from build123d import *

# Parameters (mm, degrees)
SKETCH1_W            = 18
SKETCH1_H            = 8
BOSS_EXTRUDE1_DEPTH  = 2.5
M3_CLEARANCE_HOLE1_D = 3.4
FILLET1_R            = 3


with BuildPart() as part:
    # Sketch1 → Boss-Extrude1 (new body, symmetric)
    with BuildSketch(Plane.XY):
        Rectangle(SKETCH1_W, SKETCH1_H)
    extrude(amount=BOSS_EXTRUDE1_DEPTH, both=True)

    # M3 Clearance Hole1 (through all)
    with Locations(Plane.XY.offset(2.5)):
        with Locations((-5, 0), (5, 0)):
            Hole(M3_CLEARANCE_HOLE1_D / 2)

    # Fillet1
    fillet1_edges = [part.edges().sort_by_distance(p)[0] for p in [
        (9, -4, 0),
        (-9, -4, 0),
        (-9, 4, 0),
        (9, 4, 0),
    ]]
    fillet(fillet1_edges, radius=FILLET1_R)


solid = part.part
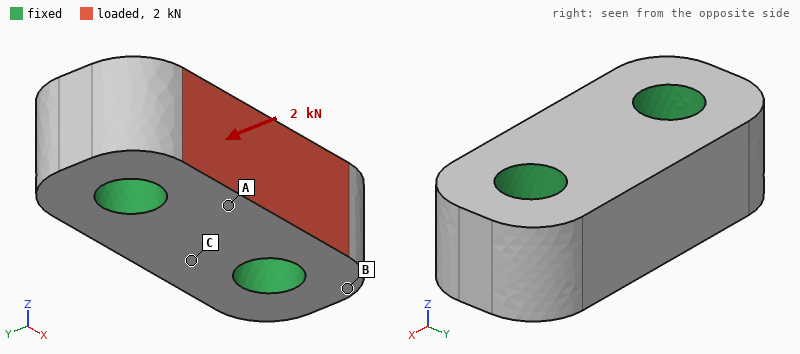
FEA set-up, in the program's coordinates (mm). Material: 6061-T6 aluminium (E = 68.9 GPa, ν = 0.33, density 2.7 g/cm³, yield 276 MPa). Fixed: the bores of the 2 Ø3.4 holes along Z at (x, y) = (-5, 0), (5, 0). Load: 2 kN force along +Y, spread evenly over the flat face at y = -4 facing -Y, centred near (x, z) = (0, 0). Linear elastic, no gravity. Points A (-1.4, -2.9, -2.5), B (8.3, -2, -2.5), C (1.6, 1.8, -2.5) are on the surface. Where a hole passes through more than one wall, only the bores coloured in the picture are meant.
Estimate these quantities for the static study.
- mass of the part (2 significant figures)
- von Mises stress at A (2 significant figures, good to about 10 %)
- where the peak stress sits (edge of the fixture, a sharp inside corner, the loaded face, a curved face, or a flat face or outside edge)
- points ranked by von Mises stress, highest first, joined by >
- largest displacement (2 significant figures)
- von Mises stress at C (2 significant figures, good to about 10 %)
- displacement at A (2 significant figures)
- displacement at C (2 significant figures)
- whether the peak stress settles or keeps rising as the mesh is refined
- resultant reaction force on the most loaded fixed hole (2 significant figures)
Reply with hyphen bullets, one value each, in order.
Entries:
- 1.6 g
- 29 MPa
- edge of the fixture
- A > C > B
- 3.0 µm
- 16 MPa
- 2.4 µm
- 1.1 µm
- keeps rising
- 1.0 kN
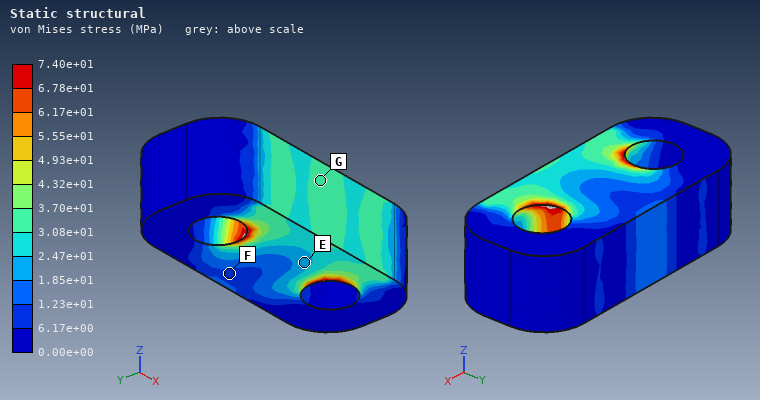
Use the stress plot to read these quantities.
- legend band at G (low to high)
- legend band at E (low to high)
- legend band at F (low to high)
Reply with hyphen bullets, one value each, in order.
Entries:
- 3.08e+01 to 3.70e+01 MPa
- 1.85e+01 to 2.47e+01 MPa
- 6.17e+00 to 1.23e+01 MPa
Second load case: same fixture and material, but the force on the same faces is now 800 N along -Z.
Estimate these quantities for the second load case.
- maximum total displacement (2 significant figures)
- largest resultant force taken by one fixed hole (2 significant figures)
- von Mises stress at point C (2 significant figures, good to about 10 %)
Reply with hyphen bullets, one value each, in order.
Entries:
- 4.9 µm
- 400 N
- 11 MPa
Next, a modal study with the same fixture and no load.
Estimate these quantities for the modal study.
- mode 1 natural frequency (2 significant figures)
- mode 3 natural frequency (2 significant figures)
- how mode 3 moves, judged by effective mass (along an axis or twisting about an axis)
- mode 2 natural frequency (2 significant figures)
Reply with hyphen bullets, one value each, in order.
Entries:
- 150 kHz
- 160 kHz
- along Y
- 150 kHz
